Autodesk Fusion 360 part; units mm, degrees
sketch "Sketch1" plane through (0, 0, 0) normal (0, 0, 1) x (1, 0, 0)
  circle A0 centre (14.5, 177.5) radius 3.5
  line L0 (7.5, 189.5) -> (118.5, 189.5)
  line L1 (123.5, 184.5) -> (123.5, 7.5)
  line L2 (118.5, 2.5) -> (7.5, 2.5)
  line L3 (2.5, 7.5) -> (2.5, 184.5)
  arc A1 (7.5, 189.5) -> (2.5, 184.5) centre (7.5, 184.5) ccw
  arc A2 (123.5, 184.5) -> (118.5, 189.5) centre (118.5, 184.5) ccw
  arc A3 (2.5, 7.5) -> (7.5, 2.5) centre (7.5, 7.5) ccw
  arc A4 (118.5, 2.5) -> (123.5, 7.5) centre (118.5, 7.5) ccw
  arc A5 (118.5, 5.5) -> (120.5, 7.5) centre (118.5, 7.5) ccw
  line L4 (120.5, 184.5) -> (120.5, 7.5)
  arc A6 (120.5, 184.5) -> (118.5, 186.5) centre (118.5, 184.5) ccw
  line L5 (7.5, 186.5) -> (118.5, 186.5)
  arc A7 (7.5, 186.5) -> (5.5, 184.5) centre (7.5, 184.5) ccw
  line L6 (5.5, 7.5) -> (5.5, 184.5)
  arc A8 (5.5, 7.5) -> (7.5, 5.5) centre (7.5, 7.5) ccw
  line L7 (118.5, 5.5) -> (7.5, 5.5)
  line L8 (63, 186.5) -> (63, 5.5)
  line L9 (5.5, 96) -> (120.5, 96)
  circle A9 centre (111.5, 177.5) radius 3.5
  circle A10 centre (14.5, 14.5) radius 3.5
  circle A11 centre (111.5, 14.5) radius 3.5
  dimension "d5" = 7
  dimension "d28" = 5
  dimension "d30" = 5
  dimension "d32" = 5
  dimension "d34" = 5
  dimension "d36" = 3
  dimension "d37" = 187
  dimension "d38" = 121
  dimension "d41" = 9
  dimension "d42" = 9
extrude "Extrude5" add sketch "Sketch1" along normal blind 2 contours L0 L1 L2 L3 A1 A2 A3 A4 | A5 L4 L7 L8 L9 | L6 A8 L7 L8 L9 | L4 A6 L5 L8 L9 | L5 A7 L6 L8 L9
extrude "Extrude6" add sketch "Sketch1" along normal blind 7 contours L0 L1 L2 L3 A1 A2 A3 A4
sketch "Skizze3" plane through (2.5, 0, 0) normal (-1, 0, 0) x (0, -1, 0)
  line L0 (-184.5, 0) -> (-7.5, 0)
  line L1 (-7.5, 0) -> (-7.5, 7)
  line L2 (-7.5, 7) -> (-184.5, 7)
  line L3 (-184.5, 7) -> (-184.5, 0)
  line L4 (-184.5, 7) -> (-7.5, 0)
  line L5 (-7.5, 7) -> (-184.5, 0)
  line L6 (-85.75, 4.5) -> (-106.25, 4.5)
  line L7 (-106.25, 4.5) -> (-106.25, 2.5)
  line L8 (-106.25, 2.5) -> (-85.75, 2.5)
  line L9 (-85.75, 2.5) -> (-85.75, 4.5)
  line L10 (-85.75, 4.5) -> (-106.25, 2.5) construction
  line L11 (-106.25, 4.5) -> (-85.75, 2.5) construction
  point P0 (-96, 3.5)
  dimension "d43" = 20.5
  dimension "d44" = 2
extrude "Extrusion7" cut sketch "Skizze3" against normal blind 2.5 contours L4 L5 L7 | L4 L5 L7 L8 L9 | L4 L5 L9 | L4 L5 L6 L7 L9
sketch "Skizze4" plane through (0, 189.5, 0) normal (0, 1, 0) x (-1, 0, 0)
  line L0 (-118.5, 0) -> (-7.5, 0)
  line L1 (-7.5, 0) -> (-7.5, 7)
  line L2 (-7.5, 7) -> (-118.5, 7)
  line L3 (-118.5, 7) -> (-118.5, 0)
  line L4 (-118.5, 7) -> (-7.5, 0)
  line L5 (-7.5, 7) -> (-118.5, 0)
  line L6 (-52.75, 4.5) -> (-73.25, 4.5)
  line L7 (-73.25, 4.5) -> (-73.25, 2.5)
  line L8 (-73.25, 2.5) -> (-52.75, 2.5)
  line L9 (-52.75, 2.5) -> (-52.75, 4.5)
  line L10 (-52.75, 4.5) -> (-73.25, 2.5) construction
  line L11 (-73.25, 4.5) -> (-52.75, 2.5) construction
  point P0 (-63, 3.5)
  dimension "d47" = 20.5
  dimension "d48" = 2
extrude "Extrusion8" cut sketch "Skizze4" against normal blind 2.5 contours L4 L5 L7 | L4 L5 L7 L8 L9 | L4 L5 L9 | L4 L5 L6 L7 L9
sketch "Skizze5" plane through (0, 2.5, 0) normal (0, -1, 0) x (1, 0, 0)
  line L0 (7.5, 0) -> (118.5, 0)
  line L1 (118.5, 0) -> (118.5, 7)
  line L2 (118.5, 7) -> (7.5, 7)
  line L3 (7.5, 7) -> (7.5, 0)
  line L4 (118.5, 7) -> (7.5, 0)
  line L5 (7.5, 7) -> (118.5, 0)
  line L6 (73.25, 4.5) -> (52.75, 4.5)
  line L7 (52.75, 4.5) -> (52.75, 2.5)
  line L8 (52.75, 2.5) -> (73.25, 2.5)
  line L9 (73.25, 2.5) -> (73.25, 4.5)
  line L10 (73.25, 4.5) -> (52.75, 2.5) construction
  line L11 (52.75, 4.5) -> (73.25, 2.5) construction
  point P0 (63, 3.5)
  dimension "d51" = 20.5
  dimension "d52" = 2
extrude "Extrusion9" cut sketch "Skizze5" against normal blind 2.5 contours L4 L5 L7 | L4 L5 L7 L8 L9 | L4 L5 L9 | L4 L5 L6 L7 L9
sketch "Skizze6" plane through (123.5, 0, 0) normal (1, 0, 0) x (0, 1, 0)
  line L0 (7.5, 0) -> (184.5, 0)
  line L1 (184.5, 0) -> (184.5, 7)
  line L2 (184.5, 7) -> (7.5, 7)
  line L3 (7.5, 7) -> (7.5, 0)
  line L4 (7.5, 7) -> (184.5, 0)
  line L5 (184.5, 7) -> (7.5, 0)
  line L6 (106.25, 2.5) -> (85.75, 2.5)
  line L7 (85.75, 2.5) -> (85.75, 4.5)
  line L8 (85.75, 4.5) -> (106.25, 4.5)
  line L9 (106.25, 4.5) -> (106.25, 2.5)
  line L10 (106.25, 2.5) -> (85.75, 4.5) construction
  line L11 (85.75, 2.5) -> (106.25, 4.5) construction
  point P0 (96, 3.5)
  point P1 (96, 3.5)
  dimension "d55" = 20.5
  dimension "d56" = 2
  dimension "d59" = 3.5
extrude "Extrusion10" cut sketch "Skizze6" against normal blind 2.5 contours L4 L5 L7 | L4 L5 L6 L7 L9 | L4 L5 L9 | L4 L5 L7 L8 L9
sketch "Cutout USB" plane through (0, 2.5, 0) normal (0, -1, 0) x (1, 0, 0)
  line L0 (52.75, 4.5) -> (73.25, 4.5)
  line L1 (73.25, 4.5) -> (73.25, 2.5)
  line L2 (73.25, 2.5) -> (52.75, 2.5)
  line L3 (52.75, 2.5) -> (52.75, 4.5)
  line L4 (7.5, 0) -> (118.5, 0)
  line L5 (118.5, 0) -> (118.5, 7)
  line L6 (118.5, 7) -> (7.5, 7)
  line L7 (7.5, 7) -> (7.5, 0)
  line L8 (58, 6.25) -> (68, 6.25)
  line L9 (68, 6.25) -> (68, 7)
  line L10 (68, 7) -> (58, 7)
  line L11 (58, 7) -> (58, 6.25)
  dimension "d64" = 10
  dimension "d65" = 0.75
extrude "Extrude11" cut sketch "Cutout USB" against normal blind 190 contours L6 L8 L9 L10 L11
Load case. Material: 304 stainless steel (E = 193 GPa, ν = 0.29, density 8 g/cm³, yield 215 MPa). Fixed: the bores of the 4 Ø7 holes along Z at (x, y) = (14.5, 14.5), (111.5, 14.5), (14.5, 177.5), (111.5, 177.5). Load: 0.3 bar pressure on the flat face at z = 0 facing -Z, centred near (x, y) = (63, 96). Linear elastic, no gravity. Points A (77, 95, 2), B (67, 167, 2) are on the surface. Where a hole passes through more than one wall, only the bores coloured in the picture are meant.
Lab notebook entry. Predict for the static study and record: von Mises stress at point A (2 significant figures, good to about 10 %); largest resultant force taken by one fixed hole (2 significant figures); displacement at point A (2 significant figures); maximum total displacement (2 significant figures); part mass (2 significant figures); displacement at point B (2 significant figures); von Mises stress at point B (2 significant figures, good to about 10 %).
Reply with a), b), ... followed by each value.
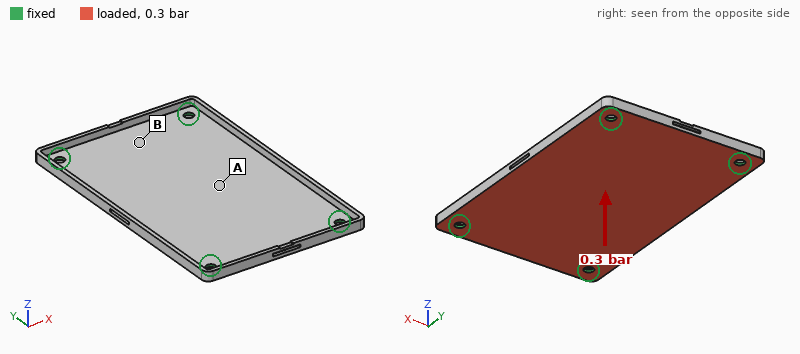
a) 29 MPa
b) 190 N
c) 0.28 mm
d) 0.29 mm
e) 430 g
f) 0.082 mm
g) 19 MPa
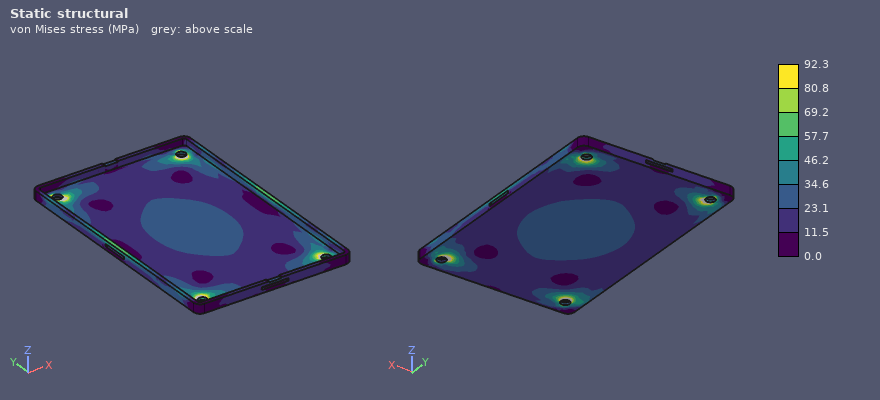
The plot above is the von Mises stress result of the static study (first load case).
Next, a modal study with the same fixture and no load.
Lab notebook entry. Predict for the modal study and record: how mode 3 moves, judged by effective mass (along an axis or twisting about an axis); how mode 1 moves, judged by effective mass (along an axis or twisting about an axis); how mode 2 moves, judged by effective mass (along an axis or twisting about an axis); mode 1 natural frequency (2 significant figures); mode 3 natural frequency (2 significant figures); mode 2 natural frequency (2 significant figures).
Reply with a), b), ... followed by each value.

a) twisting about X
b) along Z
c) twisting about Y
d) 500 Hz
e) 1100 Hz
f) 850 Hz
